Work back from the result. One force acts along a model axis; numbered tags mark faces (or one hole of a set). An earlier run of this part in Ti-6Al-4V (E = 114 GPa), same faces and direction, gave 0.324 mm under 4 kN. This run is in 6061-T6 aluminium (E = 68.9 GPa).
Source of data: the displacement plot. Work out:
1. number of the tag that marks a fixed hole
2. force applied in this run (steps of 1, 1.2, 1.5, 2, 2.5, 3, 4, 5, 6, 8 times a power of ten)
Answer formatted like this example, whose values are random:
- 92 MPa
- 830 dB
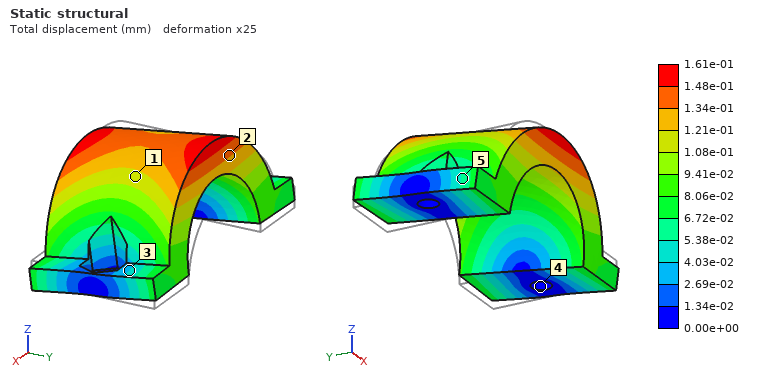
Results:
- 4
- 1.2 kN
